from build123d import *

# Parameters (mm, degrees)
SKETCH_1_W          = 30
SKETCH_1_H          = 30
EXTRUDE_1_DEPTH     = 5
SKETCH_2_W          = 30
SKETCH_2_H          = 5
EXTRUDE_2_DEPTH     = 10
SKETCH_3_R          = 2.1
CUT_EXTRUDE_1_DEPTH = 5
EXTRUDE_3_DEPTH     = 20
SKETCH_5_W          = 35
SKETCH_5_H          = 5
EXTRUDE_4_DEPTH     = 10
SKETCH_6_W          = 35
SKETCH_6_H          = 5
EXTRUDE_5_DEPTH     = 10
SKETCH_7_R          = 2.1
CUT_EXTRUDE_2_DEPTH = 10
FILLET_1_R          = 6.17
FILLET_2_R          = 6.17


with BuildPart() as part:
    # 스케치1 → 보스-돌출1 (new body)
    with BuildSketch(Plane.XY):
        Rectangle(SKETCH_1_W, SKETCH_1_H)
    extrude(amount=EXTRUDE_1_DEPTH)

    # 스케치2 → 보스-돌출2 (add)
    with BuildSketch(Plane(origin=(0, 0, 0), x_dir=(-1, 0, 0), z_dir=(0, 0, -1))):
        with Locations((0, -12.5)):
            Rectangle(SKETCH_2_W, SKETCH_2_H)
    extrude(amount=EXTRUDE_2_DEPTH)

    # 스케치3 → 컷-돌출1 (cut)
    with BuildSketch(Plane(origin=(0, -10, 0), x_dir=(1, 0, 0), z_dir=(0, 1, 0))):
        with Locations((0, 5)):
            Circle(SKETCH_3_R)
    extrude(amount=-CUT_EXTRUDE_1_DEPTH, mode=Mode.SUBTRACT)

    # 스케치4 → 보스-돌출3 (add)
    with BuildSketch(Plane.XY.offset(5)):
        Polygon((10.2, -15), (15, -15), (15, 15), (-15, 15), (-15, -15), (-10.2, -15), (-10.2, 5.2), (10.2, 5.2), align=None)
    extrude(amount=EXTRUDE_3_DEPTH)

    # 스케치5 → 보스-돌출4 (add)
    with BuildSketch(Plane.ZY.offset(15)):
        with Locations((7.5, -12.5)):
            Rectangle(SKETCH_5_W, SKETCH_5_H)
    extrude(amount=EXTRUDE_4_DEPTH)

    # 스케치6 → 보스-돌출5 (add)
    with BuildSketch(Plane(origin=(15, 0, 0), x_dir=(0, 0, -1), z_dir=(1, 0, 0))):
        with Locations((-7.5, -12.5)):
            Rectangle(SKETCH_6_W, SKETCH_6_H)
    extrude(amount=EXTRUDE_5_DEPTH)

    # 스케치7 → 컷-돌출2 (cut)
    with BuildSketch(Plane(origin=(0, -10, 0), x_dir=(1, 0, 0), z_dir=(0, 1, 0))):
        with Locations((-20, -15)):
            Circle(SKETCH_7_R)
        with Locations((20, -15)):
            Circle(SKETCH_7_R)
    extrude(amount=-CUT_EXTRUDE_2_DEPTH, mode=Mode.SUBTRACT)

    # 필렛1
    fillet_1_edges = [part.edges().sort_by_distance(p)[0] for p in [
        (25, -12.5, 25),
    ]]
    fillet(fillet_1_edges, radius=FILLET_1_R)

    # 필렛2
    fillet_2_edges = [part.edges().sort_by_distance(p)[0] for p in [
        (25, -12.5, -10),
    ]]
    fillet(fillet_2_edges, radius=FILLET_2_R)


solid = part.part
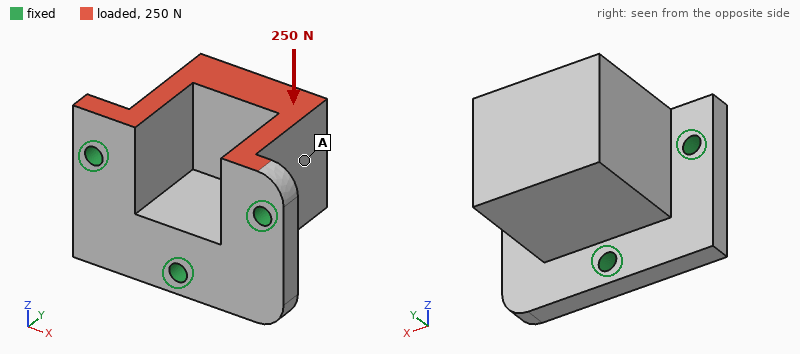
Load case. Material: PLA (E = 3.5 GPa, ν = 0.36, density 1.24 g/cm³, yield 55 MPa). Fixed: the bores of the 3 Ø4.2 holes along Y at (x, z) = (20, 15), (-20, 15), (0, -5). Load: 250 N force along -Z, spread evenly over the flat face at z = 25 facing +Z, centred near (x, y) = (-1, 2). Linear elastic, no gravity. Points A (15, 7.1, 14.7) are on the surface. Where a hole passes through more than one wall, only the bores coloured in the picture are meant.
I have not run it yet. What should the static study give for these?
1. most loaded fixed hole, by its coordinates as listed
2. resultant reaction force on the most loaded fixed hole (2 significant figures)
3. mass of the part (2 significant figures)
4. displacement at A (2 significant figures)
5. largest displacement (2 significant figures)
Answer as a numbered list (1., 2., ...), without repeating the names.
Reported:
1. (0, -5)
2. 180 N
3. 24 g
4. 61 µm
5. 91 µm
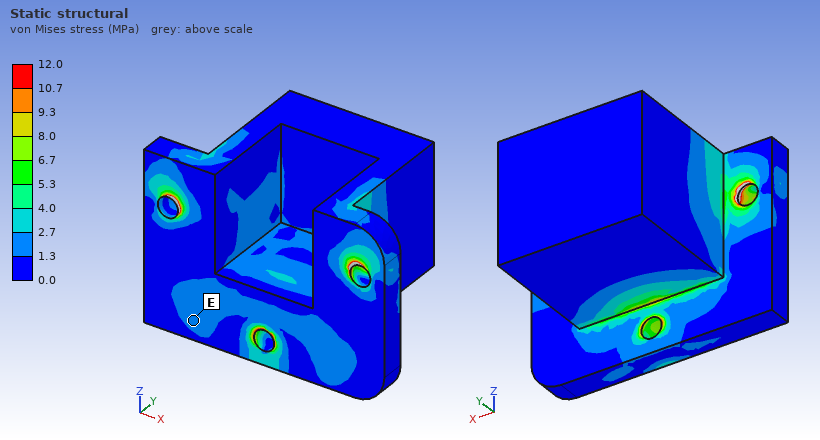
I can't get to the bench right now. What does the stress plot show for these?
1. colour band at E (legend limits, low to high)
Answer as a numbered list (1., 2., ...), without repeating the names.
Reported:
1. 1.3 to 2.7 MPa
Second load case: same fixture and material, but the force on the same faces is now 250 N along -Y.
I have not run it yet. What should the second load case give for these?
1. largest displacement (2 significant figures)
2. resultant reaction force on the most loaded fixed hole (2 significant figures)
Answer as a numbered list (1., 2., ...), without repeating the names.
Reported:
1. 0.11 mm
2. 180 N
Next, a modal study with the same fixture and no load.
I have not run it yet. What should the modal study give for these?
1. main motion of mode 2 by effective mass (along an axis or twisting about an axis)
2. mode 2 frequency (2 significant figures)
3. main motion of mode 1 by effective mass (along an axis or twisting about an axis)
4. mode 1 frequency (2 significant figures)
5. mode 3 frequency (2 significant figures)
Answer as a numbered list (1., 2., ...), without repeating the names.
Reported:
1. along X
2. 2400 Hz
3. along Z
4. 2200 Hz
5. 4300 Hz
